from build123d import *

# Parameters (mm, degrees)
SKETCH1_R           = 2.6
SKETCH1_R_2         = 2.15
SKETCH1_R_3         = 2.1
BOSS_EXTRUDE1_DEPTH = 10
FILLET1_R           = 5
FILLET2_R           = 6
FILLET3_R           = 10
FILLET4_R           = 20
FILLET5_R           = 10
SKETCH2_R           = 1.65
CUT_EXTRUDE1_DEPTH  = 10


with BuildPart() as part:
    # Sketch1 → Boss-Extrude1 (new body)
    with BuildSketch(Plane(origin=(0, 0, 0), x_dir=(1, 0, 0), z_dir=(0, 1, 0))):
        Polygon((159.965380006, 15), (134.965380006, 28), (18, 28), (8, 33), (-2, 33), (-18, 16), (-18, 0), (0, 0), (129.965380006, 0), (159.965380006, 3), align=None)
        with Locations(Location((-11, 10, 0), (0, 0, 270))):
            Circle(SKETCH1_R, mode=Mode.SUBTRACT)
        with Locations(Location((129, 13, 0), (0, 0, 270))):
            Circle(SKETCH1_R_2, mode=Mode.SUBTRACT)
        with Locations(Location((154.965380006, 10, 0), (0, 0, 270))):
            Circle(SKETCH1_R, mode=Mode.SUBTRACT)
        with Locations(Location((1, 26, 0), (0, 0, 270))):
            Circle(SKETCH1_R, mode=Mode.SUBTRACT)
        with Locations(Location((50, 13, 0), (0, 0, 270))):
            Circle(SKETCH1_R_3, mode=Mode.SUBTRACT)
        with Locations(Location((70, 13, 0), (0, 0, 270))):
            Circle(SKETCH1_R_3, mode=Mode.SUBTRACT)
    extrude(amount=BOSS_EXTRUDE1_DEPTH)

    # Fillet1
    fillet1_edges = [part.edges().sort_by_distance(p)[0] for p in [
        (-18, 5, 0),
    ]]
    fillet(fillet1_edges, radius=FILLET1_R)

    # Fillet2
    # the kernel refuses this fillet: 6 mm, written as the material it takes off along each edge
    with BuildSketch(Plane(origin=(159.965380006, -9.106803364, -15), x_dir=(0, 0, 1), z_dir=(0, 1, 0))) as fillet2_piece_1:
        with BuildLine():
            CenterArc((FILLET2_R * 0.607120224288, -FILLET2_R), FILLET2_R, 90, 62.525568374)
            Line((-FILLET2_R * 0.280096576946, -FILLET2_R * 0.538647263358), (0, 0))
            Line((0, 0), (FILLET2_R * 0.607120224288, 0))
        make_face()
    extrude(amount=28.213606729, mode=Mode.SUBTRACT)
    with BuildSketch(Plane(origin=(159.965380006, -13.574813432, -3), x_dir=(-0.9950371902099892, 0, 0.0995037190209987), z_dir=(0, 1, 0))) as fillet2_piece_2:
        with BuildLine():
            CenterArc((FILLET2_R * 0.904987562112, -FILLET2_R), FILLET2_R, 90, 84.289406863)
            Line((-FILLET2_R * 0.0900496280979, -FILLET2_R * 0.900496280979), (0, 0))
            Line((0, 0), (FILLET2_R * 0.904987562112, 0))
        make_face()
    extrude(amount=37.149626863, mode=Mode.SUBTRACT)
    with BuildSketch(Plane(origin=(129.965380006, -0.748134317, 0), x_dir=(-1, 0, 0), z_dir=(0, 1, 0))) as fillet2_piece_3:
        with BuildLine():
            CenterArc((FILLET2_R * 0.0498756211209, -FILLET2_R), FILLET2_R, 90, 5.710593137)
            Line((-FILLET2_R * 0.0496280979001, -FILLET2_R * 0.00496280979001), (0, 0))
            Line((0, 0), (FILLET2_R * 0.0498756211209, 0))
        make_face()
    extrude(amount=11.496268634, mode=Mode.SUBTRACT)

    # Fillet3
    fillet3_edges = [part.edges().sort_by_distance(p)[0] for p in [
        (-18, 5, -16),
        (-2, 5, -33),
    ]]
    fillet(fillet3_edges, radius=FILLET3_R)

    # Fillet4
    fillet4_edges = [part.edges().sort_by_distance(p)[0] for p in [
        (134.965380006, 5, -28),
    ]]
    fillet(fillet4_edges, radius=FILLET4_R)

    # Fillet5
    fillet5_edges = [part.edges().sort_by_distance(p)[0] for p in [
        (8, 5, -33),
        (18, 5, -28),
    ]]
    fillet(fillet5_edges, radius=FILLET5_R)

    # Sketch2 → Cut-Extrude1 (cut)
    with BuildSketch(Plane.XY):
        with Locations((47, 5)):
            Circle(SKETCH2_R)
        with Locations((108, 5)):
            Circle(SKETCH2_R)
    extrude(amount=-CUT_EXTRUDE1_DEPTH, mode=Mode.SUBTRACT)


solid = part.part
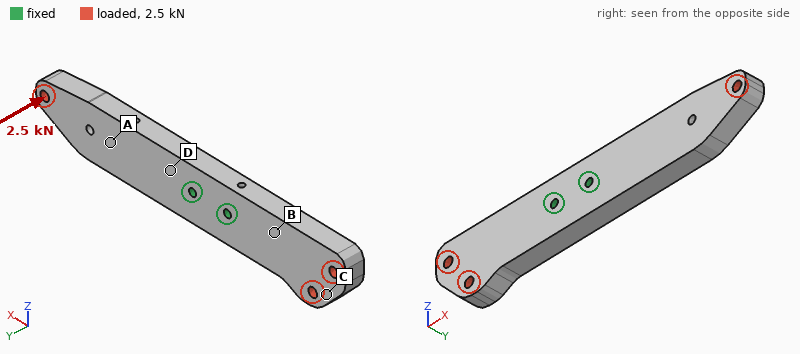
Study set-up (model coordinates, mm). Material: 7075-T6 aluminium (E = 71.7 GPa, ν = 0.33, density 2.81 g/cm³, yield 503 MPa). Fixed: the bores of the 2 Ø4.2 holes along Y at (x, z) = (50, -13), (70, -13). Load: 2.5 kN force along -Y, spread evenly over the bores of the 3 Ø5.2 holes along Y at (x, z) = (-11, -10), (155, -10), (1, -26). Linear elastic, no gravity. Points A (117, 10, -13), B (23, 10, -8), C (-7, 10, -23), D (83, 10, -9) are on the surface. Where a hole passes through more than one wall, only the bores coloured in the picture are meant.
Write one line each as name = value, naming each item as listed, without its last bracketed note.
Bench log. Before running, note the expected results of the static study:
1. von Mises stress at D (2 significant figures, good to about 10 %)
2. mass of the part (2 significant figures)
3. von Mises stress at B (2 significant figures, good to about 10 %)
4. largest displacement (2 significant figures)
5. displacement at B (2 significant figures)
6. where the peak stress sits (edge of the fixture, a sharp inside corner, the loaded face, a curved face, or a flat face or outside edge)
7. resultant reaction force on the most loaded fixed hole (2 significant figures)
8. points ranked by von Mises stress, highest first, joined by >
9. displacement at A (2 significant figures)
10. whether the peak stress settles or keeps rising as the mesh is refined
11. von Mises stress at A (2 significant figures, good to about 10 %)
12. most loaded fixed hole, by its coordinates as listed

von Mises stress at D = 130 MPa
mass of the part = 130 g
von Mises stress at B = 98 MPa
largest displacement = 1.2 mm
displacement at B = 0.21 mm
where the peak stress sits = edge of the fixture
resultant reaction force on the most loaded fixed hole = 2.1 kN
points ranked by von Mises stress, highest first, joined by > = D > B > A > C
displacement at A = 0.44 mm
whether the peak stress settles or keeps rising as the mesh is refined = keeps rising
von Mises stress at A = 66 MPa
most loaded fixed hole, by its coordinates as listed = (50, -13)
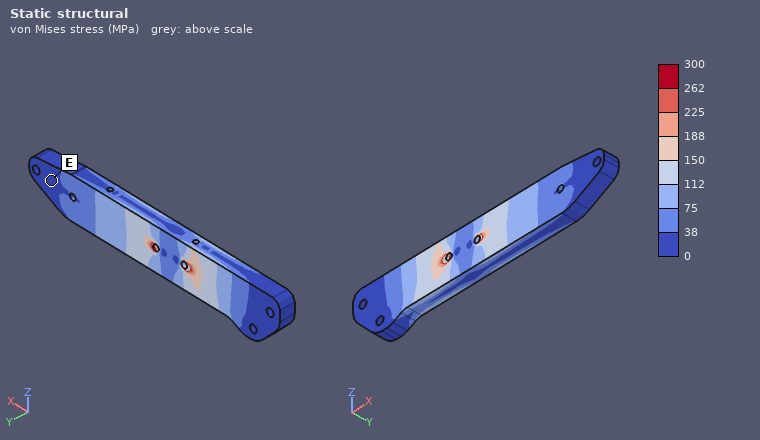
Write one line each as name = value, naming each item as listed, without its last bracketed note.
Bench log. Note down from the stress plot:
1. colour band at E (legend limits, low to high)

colour band at E = 0 to 38 MPa
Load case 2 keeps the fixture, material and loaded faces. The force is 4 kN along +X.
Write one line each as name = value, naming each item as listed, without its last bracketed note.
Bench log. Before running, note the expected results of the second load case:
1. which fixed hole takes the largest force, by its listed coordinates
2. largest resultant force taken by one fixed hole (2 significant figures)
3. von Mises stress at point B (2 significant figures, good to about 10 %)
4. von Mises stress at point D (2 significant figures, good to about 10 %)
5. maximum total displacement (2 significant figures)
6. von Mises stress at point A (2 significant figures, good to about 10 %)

which fixed hole takes the largest force, by its listed coordinates = (50, -13)
largest resultant force taken by one fixed hole = 2.3 kN
von Mises stress at point B = 6.3 MPa
von Mises stress at point D = 7.6 MPa
maximum total displacement = 26 µm
von Mises stress at point A = 4.8 MPa
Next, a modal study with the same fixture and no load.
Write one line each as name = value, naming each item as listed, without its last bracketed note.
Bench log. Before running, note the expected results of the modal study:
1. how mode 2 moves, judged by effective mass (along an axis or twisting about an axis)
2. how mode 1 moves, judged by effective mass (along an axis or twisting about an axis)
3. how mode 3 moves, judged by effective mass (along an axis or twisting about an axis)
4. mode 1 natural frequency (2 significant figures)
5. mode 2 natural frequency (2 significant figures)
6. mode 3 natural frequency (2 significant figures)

how mode 2 moves, judged by effective mass = along Y
how mode 1 moves, judged by effective mass = along Y
how mode 3 moves, judged by effective mass = along Z
mode 1 natural frequency = 1100 Hz
mode 2 natural frequency = 1800 Hz
mode 3 natural frequency = 2400 Hz
